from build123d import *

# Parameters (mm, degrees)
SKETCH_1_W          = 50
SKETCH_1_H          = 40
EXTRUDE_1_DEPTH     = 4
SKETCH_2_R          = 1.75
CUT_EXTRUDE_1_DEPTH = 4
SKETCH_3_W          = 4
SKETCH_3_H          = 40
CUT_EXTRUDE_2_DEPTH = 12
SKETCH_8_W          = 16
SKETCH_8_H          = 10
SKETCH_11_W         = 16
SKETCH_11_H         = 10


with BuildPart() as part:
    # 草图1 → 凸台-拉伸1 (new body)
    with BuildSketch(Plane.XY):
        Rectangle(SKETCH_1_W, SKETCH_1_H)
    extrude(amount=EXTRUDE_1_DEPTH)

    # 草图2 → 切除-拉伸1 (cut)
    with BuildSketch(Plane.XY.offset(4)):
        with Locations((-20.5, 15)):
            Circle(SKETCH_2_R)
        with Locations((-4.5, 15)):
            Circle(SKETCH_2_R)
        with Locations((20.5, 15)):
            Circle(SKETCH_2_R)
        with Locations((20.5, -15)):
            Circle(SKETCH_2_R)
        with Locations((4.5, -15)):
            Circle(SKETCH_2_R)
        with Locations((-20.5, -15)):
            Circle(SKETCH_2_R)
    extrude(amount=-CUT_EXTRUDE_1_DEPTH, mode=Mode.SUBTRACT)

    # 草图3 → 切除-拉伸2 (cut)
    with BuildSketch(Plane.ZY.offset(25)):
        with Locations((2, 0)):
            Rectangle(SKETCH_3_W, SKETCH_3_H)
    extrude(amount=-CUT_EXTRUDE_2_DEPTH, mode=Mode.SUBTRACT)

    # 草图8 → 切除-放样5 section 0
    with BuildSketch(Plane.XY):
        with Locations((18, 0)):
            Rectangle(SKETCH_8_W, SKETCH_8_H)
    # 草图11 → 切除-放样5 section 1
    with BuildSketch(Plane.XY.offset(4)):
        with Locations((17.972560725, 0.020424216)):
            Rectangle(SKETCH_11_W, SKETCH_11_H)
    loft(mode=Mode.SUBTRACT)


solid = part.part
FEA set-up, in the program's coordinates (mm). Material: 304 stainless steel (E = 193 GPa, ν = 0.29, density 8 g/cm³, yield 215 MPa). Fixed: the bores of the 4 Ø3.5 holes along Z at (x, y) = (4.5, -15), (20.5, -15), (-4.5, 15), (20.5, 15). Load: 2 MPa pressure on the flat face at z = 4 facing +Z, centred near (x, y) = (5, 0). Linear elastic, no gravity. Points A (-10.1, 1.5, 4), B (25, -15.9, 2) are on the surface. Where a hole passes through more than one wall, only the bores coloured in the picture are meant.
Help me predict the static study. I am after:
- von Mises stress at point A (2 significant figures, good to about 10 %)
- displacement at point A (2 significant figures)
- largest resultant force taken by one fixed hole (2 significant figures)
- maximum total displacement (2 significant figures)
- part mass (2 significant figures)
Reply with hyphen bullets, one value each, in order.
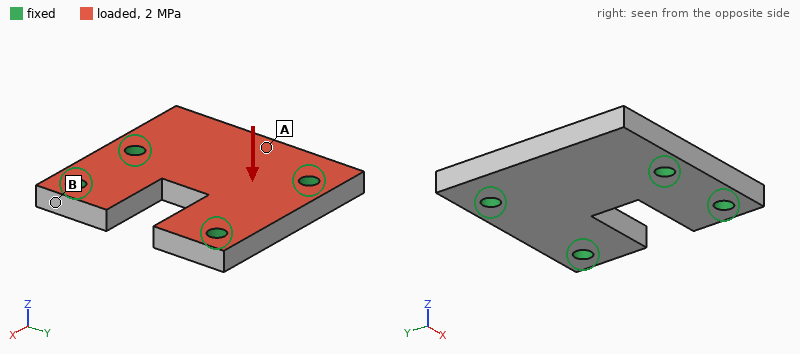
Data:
- 32 MPa
- 12 µm
- 980 N
- 20 µm
- 43 g
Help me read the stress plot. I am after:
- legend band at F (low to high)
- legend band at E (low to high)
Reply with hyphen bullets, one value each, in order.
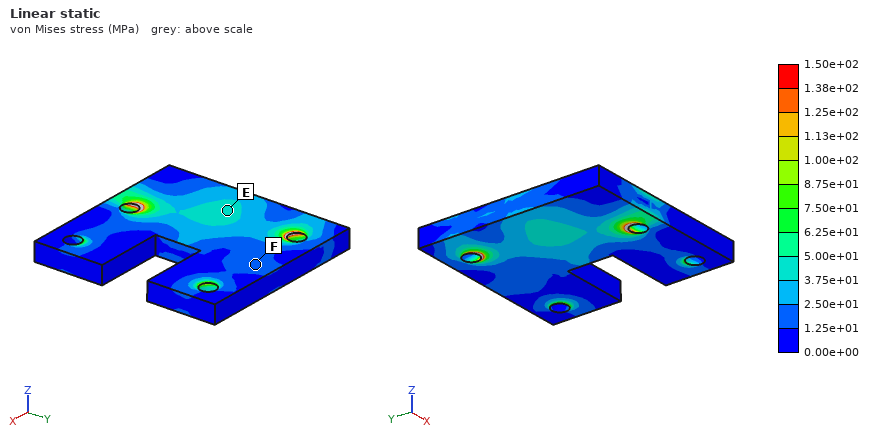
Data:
- 1.25e+01 to 2.50e+01 MPa
- 3.75e+01 to 5.00e+01 MPa
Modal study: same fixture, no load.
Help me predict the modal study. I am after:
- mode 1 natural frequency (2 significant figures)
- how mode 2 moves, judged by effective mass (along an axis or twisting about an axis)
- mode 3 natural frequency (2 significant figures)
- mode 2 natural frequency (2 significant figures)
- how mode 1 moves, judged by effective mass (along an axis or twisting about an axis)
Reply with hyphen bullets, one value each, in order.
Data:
- 11 kHz
- along Z
- 24 kHz
- 19 kHz
- along Z
